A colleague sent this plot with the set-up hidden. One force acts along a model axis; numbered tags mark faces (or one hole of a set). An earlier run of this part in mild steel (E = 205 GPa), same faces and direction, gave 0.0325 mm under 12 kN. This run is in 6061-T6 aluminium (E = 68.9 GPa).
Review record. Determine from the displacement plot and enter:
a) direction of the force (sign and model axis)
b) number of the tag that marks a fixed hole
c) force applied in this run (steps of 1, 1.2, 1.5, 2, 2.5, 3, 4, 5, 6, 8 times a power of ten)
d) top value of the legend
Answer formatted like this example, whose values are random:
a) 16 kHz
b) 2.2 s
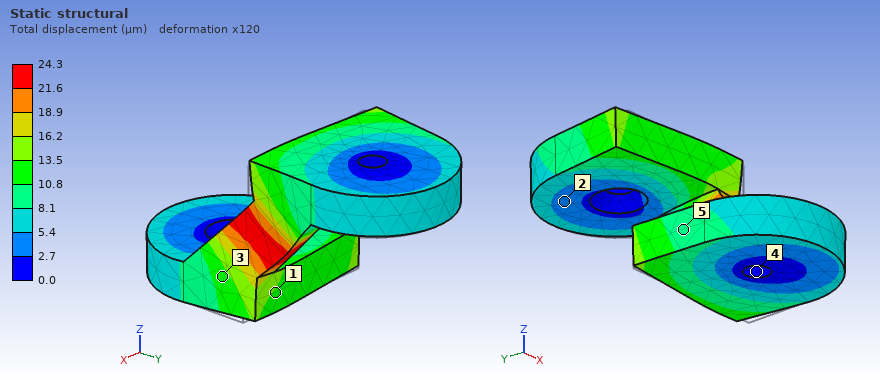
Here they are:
a) -X
b) 4
c) 3 kN
d) 24.3 µm
